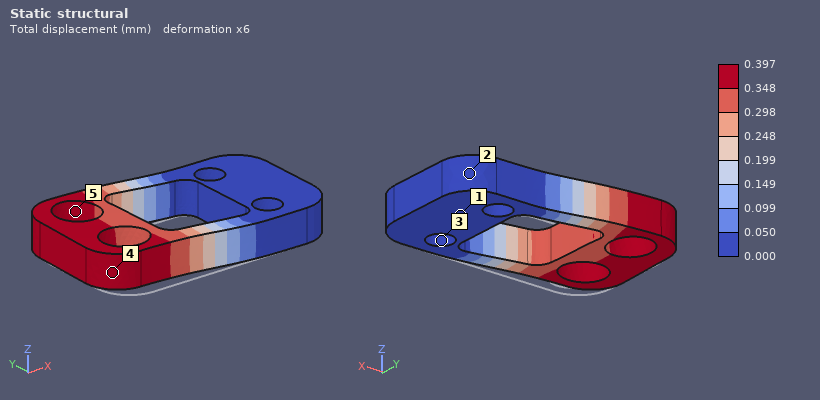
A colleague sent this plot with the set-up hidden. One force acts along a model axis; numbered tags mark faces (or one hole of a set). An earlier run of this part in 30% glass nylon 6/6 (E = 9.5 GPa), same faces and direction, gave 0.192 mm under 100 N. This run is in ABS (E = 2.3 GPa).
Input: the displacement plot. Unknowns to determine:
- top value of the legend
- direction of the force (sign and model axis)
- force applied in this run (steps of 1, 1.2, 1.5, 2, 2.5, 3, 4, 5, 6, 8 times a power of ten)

0.397 mm
+Y
50 N
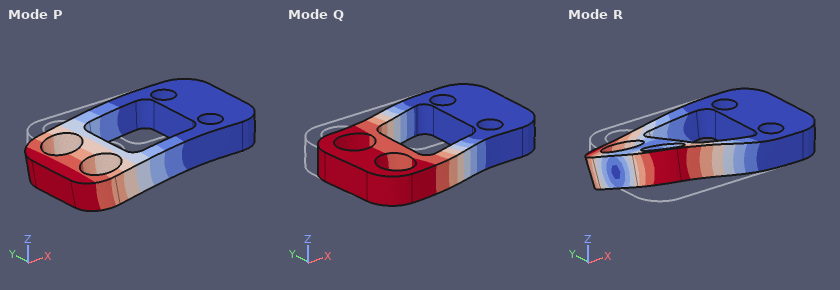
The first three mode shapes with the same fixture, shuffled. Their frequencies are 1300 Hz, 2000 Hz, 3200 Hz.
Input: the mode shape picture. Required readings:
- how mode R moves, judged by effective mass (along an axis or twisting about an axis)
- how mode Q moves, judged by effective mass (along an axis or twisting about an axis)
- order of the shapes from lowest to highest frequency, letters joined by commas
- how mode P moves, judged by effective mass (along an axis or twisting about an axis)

twisting about X
along Y
P, Q, R
along Z
